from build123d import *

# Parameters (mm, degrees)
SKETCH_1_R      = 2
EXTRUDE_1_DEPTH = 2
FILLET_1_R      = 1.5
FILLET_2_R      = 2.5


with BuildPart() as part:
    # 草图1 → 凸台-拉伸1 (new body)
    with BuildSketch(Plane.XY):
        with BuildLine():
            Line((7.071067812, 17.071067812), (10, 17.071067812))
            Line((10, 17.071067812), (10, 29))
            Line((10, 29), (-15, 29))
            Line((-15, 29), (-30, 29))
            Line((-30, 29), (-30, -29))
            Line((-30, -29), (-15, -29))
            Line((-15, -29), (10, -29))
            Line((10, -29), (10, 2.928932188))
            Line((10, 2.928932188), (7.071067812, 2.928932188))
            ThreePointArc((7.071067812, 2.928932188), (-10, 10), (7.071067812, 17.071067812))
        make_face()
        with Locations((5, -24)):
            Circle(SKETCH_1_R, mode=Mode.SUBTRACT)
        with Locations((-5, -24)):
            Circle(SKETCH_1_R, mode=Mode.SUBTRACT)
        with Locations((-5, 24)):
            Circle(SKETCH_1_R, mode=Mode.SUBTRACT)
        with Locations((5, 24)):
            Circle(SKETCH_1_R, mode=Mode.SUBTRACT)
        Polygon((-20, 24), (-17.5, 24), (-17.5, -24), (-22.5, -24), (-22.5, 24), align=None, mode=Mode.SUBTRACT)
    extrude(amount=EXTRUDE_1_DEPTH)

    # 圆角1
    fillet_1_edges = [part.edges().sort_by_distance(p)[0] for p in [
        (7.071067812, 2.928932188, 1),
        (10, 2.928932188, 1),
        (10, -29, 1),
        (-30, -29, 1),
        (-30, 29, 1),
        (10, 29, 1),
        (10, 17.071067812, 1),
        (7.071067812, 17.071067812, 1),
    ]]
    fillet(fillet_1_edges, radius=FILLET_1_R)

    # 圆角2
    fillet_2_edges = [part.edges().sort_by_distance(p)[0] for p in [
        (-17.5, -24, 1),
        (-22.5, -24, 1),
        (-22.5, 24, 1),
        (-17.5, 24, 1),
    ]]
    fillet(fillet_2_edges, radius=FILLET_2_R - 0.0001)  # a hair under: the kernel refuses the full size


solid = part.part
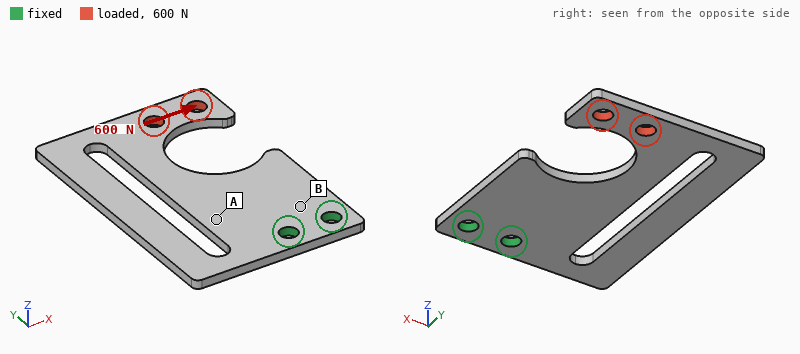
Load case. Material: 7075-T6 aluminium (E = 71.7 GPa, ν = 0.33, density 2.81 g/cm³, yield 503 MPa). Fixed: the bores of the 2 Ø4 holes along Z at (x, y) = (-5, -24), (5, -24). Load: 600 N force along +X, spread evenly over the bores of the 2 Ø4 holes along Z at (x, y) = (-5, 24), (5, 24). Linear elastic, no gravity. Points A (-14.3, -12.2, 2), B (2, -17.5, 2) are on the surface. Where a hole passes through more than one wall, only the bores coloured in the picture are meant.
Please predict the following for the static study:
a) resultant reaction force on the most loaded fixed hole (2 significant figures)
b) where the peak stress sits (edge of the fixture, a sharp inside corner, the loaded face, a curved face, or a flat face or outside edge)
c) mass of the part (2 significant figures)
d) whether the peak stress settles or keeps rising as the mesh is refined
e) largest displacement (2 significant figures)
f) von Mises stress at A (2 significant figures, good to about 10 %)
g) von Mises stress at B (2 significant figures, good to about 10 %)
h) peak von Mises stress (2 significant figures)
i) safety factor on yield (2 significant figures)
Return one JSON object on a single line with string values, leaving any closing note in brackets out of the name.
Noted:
{"resultant reaction force on the most loaded fixed hole": "2.1 kN", "where the peak stress sits": "a curved face", "mass of the part": "9.6 g", "whether the peak stress settles or keeps rising as the mesh is refined": "settles", "largest displacement": "0.63 mm", "von Mises stress at A": "50 MPa", "von Mises stress at B": "100 MPa", "peak von Mises stress": "410 MPa", "safety factor on yield": "1.2"}
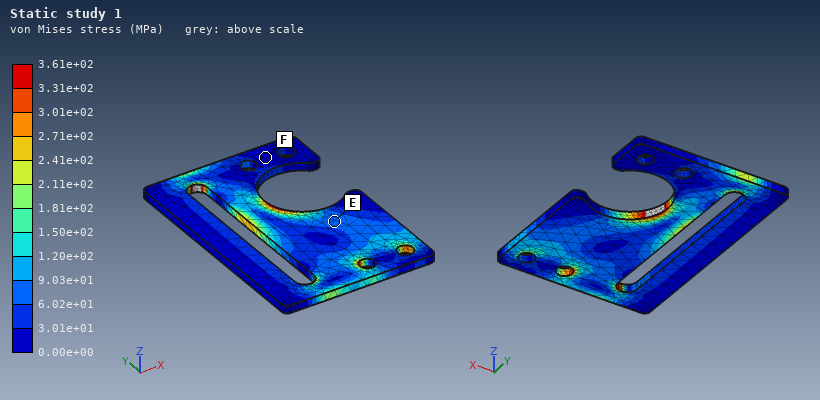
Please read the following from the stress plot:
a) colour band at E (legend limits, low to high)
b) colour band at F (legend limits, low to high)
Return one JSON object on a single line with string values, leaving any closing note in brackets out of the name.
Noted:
{"colour band at E": "6.02e+01 to 9.03e+01 MPa", "colour band at F": "0.00e+00 to 3.01e+01 MPa"}
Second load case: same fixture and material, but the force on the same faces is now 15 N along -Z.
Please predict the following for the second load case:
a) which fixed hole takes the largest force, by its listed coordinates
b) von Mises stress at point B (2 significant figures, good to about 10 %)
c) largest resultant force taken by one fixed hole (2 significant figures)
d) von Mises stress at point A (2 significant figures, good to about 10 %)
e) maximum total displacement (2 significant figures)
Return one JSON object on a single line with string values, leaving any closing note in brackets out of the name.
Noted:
{"which fixed hole takes the largest force, by its listed coordinates": "(-5, -24)", "von Mises stress at point B": "30 MPa", "largest resultant force taken by one fixed hole": "13 N", "von Mises stress at point A": "27 MPa", "maximum total displacement": "0.75 mm"}
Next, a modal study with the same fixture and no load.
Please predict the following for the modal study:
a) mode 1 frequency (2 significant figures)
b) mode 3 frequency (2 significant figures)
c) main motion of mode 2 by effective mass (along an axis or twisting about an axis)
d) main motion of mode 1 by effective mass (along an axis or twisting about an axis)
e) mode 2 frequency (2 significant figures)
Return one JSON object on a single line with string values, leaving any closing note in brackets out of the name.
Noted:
{"mode 1 frequency": "530 Hz", "mode 3 frequency": "2400 Hz", "main motion of mode 2 by effective mass": "twisting about Y", "main motion of mode 1 by effective mass": "along Z", "mode 2 frequency": "1100 Hz"}
